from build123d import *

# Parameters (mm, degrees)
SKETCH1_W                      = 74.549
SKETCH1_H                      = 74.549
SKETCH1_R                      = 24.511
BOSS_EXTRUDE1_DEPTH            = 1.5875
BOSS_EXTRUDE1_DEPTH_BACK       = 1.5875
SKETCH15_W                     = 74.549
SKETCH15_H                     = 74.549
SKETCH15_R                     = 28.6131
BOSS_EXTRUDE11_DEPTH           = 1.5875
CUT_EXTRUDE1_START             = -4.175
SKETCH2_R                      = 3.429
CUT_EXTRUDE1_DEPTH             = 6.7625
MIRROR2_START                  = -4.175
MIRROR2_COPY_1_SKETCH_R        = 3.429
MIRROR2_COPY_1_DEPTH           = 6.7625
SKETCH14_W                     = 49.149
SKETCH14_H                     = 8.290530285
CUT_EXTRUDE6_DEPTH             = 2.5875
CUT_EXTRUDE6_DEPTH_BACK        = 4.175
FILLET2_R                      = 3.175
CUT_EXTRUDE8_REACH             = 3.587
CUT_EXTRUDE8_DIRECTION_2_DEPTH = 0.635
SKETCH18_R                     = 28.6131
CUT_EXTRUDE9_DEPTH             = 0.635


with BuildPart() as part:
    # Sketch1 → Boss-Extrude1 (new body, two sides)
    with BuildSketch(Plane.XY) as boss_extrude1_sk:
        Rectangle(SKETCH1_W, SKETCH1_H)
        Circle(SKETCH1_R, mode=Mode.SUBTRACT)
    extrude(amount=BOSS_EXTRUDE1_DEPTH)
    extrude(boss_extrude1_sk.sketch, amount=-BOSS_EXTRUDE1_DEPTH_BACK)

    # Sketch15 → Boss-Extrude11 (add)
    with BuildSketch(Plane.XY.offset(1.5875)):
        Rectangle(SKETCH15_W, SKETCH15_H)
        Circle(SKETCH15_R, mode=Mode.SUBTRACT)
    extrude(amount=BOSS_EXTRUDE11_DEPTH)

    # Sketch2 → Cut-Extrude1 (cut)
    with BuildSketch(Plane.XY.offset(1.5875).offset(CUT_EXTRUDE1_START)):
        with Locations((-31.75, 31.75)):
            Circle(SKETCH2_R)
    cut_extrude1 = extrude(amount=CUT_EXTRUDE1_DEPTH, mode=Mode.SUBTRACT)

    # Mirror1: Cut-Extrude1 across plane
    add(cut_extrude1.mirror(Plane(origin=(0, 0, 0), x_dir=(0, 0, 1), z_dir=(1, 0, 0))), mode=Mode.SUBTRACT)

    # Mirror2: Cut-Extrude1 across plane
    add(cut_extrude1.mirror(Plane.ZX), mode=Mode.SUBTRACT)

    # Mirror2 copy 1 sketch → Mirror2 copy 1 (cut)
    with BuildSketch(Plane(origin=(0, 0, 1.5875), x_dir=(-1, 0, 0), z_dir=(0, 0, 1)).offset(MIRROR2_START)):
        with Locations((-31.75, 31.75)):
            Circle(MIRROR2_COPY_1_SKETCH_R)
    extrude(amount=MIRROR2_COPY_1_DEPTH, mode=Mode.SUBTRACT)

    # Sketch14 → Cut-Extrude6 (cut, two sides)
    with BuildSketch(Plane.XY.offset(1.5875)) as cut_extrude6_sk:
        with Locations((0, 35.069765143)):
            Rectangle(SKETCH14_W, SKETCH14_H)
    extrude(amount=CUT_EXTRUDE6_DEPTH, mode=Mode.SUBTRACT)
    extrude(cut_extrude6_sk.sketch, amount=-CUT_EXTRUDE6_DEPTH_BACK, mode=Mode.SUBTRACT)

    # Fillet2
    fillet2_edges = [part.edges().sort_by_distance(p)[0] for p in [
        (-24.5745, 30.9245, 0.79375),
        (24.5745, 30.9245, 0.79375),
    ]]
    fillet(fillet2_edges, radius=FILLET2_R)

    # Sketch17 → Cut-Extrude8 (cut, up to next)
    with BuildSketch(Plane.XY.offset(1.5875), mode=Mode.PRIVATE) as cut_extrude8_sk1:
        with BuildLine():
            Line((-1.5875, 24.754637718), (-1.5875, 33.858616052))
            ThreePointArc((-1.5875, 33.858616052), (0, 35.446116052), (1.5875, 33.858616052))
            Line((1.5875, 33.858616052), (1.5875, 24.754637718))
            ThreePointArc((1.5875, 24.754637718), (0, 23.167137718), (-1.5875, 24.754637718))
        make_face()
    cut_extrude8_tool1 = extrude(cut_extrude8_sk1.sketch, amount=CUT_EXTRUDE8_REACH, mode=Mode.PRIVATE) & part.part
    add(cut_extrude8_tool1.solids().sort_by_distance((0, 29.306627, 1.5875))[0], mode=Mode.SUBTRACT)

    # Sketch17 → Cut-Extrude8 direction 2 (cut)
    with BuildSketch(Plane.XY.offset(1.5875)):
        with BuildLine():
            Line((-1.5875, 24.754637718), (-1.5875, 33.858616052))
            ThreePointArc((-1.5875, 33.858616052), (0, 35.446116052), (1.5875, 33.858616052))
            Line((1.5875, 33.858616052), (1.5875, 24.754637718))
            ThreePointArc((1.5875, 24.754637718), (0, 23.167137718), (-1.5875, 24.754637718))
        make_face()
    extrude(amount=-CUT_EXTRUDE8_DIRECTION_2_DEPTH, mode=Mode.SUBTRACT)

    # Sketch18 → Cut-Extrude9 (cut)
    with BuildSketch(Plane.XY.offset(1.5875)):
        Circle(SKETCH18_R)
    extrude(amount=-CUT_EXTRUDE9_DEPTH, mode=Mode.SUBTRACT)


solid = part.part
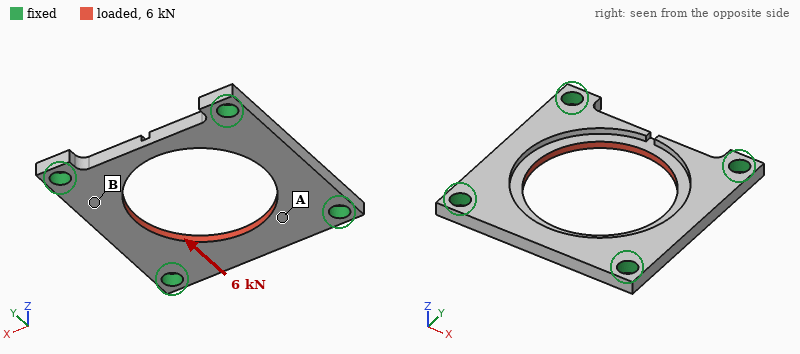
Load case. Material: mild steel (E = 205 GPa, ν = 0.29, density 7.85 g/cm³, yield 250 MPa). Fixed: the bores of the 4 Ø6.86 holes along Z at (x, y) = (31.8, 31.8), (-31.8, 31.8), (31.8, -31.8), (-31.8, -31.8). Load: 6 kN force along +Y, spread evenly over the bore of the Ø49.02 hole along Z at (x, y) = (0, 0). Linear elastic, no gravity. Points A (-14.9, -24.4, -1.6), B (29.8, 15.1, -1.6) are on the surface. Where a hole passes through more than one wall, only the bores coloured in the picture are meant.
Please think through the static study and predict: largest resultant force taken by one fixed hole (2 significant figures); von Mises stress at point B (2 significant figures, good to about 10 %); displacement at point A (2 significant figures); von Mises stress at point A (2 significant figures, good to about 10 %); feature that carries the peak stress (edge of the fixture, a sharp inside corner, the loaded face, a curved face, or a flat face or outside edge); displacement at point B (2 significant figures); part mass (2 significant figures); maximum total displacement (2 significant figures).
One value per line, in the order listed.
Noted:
1.5 kN
13 MPa
4.7 µm
28 MPa
a flat face or outside edge
2.9 µm
110 g
18 µm
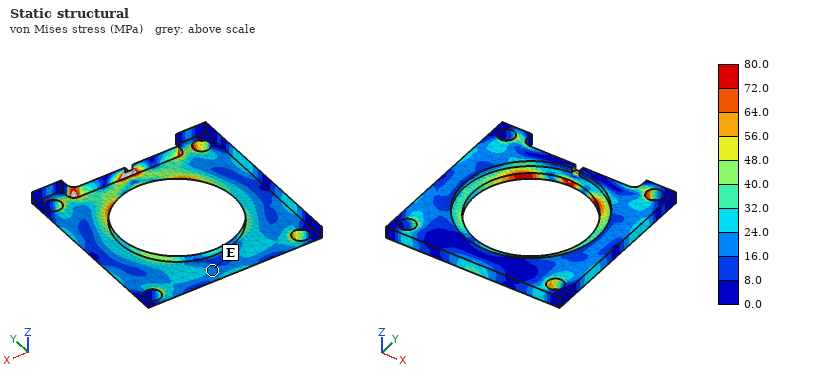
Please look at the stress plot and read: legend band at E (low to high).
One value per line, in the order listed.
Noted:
16.0 to 24.0 MPa
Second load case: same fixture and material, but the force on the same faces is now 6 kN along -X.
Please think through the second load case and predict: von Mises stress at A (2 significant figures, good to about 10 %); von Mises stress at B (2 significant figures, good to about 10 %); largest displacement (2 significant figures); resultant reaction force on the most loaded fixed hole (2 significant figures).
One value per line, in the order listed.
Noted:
25 MPa
29 MPa
12 µm
1.6 kN
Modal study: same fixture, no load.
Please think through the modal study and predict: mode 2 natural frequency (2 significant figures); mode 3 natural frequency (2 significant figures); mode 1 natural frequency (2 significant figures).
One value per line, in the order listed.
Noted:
7300 Hz
7300 Hz
7200 Hz
